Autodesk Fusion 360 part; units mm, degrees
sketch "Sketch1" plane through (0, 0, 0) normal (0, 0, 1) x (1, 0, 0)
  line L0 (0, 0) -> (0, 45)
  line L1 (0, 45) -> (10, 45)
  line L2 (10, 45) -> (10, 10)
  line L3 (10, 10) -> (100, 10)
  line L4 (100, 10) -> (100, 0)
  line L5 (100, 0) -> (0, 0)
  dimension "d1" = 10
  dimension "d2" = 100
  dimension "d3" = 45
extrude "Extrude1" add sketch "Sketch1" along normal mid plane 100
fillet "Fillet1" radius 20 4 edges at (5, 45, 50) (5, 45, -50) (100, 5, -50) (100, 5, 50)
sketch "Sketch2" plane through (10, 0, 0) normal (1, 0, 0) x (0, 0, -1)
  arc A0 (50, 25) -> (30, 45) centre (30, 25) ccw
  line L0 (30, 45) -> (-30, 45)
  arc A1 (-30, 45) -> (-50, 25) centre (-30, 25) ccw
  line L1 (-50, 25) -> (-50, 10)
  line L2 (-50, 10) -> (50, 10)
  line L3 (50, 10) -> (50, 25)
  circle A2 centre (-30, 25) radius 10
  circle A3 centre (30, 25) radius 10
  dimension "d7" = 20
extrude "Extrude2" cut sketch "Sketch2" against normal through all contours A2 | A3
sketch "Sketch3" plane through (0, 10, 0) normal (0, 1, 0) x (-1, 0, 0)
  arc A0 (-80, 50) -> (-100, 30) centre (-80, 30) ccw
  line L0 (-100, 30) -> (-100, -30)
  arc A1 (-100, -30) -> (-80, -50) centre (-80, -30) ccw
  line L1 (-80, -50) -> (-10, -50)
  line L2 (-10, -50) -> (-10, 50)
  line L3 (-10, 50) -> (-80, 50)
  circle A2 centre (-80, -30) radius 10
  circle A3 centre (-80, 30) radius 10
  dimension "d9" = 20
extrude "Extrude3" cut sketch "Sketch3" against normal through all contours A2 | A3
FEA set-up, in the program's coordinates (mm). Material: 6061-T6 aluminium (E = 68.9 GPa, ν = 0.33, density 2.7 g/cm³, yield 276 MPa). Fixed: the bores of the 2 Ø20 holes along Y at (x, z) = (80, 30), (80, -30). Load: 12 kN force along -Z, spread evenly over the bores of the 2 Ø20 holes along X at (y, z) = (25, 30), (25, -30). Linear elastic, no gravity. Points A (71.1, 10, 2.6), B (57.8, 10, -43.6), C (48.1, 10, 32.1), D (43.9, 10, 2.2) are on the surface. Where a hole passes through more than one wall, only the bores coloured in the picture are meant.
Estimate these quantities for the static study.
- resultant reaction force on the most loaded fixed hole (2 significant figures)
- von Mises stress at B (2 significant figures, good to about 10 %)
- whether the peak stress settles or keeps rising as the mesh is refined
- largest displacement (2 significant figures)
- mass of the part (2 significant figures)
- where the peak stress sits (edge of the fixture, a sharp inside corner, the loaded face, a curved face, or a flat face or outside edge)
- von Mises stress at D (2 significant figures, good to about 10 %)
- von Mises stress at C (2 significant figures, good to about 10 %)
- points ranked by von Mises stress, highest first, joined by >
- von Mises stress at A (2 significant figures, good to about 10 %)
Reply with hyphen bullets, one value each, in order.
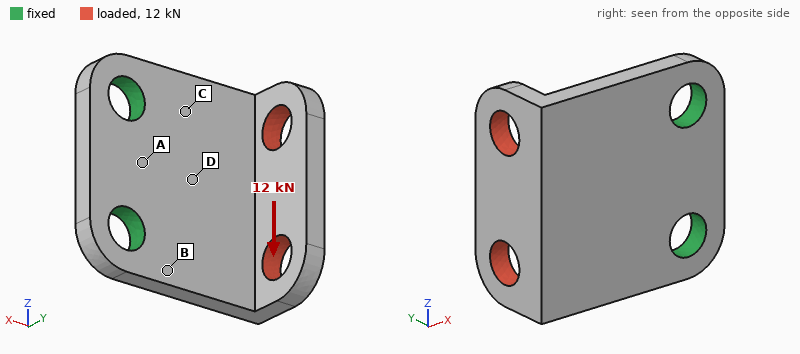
- 14 kN
- 70 MPa
- keeps rising
- 0.66 mm
- 320 g
- edge of the fixture
- 110 MPa
- 91 MPa
- D > C > B > A
- 34 MPa
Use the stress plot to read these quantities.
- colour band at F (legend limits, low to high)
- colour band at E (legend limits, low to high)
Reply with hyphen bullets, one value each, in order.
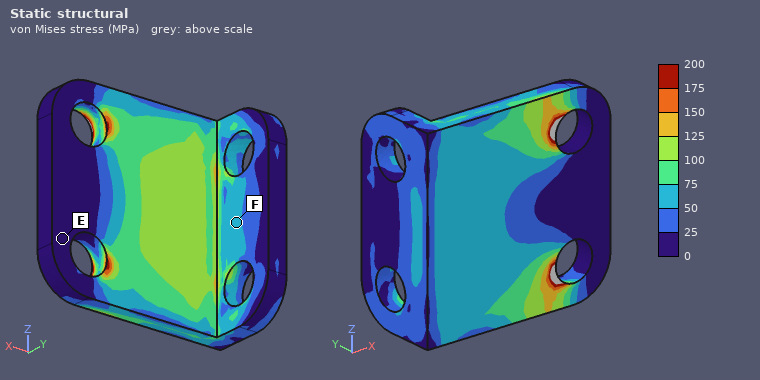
- 50 to 75 MPa
- 0 to 25 MPa
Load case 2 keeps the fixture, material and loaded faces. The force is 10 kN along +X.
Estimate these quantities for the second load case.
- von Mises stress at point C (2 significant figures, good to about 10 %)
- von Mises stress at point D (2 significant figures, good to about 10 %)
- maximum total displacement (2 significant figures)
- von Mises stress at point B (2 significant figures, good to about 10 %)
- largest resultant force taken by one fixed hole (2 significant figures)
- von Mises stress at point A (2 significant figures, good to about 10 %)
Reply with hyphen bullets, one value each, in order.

- 120 MPa
- 110 MPa
- 1.4 mm
- 130 MPa
- 5.1 kN
- 71 MPa
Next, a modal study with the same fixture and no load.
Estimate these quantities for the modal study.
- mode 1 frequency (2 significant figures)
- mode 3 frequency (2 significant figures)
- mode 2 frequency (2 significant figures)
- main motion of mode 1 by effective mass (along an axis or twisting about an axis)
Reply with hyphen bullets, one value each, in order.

- 950 Hz
- 3400 Hz
- 1900 Hz
- along Y
